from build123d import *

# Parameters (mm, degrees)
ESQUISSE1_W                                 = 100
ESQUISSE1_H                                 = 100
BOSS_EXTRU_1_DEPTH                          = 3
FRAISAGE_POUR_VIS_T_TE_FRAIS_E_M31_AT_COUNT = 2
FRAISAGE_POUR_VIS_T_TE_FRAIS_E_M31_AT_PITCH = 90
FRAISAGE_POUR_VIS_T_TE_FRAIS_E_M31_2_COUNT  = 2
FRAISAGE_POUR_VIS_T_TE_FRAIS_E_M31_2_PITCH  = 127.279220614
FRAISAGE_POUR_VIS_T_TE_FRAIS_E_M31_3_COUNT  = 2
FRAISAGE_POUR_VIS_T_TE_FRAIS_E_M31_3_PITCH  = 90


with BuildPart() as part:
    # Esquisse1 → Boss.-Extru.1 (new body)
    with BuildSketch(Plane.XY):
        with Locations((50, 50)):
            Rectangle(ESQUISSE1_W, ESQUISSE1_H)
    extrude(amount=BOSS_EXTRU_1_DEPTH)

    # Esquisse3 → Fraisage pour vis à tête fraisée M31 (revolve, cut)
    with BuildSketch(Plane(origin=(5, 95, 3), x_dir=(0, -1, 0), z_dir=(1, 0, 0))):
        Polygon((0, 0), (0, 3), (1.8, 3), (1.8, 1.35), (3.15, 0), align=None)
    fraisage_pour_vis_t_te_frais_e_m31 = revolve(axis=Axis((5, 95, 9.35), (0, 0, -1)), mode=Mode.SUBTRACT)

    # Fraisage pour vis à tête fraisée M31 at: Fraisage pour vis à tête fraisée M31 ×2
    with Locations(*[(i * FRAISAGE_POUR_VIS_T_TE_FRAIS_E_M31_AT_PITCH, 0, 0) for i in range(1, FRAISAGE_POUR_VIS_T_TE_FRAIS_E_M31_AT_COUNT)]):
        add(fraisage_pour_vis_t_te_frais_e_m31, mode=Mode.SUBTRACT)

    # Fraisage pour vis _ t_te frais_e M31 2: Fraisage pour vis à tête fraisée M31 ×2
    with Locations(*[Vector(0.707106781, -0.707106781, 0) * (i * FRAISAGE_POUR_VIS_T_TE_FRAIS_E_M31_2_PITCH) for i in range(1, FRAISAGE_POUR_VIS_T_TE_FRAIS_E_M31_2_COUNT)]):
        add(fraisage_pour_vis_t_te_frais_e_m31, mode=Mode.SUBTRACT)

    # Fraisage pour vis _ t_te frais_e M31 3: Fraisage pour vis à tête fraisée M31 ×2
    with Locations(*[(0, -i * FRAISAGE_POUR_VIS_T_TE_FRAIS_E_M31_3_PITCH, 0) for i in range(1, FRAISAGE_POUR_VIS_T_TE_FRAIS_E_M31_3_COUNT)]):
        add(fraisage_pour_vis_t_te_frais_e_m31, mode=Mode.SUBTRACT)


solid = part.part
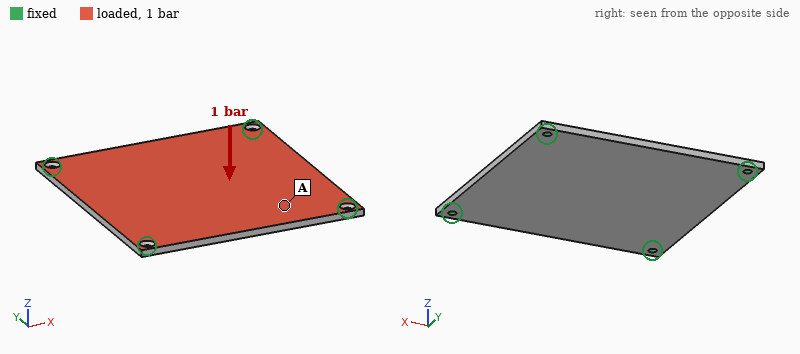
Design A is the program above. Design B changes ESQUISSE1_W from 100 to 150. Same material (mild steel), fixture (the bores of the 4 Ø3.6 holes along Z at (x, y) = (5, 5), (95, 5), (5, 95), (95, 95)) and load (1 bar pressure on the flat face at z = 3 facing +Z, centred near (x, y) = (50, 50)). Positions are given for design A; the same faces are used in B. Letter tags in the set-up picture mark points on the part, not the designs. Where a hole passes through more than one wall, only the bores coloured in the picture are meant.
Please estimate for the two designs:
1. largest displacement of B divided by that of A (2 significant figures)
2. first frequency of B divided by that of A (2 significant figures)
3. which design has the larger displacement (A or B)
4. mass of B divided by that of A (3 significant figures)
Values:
0.86
1.0
A
1.50
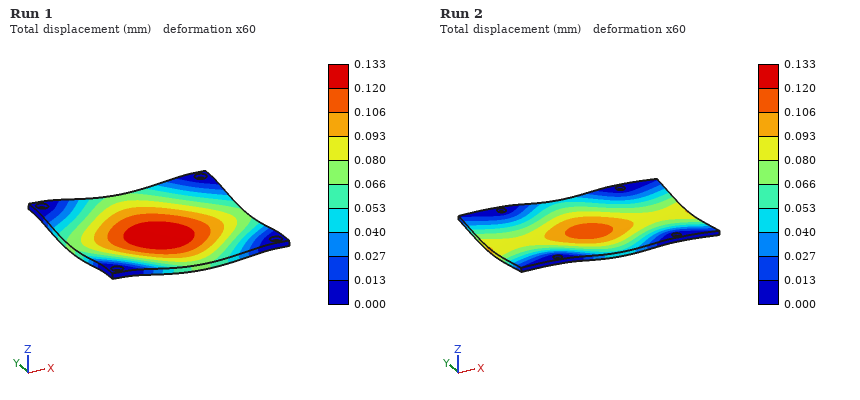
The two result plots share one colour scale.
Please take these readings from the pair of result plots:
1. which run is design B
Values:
Run 2
